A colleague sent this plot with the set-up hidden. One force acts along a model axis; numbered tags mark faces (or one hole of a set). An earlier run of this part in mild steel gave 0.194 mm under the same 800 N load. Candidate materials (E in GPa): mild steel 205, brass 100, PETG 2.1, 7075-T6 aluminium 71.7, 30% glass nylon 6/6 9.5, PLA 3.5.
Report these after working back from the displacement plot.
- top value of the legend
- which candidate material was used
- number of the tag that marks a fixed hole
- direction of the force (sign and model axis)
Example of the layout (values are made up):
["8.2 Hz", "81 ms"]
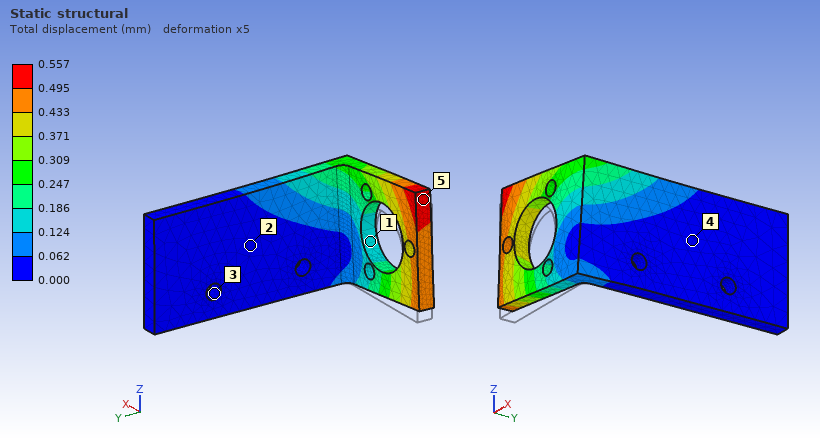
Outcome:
["0.557 mm", "7075-T6 aluminium", "3", "+Z"]
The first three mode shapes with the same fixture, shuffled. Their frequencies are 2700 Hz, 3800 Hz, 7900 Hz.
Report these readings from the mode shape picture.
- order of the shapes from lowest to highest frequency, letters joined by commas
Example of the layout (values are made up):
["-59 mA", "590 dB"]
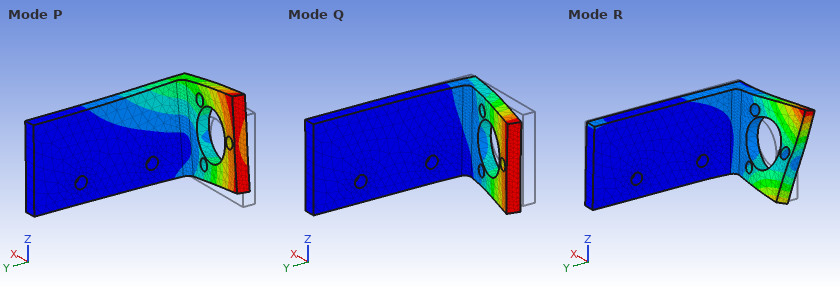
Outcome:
["Q, P, R"]
